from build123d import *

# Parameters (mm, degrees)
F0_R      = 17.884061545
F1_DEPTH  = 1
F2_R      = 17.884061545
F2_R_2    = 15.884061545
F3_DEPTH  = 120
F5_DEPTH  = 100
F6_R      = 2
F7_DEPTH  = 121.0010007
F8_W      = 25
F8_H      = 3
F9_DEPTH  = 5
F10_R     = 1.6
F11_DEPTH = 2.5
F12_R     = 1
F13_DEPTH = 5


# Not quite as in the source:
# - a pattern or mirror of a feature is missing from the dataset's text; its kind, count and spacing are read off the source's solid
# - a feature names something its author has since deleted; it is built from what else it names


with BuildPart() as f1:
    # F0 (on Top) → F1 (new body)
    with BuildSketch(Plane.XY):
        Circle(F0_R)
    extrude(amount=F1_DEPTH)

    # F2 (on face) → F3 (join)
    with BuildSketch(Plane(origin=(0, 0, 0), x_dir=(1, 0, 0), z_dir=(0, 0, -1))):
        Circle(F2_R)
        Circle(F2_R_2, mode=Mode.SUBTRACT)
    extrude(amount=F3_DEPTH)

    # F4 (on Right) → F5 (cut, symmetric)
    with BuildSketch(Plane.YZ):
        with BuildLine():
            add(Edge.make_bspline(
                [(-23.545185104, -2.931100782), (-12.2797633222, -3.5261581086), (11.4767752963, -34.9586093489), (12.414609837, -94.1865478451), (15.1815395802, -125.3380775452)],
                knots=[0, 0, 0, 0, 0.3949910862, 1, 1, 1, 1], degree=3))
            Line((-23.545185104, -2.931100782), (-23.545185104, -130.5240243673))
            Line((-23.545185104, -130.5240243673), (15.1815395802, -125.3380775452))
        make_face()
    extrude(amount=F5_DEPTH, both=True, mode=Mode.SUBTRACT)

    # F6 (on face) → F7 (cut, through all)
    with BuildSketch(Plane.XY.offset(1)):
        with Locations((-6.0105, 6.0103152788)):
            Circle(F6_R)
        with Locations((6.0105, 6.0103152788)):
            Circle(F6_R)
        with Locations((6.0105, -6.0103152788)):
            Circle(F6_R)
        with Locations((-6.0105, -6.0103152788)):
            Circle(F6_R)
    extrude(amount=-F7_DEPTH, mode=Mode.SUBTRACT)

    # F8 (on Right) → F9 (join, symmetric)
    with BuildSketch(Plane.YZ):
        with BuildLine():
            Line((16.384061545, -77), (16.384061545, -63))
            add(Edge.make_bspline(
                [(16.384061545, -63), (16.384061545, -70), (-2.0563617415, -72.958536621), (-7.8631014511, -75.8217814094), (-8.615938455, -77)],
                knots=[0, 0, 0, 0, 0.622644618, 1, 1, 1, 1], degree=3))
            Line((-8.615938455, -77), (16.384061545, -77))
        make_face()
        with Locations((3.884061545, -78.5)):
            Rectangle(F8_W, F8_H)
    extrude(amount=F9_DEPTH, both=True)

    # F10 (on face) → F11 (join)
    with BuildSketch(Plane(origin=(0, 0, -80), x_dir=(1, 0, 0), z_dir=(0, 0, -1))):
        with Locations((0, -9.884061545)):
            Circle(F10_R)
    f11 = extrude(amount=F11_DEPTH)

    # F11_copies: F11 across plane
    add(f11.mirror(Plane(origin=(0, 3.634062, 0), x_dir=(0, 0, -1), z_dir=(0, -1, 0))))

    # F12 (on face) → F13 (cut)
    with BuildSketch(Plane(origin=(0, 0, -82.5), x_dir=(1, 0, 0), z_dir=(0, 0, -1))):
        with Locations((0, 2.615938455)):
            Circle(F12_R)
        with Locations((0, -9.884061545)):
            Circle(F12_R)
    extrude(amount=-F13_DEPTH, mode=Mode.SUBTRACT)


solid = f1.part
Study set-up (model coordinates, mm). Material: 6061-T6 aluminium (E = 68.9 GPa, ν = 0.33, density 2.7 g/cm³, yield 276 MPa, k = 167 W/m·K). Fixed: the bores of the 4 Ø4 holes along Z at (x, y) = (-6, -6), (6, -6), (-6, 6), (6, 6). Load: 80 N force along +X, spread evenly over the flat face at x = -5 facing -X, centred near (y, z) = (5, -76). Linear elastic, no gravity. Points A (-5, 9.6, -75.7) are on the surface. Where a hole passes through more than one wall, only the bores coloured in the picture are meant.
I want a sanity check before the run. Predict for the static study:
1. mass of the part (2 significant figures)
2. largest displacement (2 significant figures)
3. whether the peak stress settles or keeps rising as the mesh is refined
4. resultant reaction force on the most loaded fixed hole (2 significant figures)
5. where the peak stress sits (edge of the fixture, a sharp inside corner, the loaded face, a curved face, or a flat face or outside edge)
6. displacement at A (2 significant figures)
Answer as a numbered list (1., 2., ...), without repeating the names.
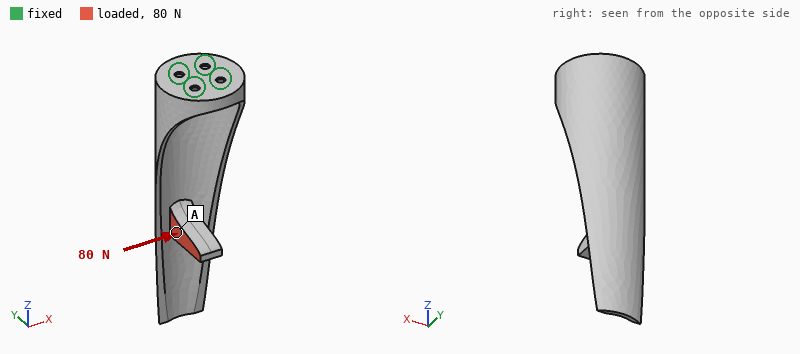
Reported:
1. 34 g
2. 0.97 mm
3. keeps rising
4. 210 N
5. edge of the fixture
6. 0.65 mm
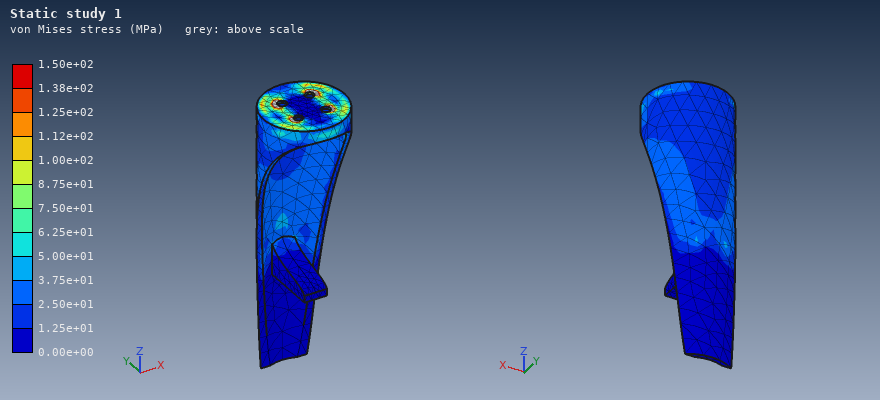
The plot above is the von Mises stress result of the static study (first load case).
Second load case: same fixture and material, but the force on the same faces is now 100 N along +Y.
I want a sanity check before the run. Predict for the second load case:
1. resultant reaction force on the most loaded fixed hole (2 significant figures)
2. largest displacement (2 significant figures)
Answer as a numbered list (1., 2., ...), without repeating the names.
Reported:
1. 230 N
2. 1.3 mm
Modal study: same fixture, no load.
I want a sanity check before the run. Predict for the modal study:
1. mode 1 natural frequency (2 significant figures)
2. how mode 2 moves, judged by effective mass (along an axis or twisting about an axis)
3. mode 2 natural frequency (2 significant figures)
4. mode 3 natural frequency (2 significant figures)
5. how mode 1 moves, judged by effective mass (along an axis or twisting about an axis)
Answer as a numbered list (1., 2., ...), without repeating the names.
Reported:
1. 420 Hz
2. along X
3. 440 Hz
4. 1500 Hz
5. along Y
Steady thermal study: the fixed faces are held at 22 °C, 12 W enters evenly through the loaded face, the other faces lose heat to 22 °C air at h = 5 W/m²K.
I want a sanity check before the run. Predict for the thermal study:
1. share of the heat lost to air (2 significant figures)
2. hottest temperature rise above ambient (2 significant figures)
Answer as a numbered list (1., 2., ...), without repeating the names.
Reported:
1. 16 %
2. 70 K
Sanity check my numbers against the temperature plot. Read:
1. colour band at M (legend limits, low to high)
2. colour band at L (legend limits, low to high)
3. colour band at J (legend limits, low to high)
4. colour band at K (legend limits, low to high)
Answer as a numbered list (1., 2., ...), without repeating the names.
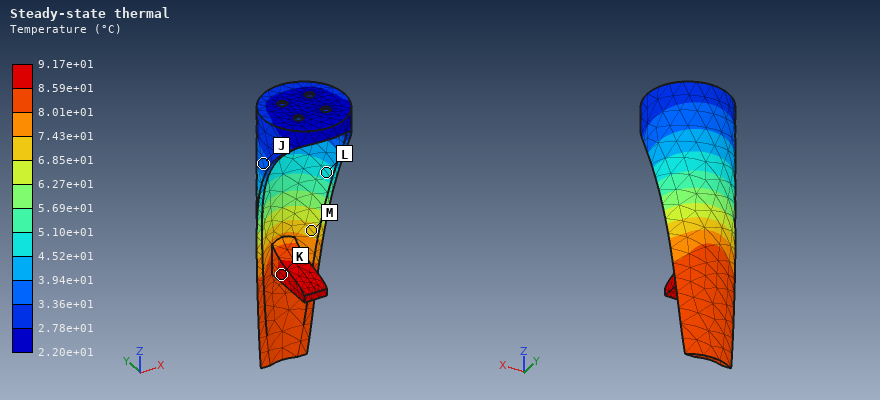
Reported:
1. 6.85e+01 to 7.43e+01 °C
2. 4.52e+01 to 5.10e+01 °C
3. 3.36e+01 to 3.94e+01 °C
4. 8.59e+01 to 9.17e+01 °C
